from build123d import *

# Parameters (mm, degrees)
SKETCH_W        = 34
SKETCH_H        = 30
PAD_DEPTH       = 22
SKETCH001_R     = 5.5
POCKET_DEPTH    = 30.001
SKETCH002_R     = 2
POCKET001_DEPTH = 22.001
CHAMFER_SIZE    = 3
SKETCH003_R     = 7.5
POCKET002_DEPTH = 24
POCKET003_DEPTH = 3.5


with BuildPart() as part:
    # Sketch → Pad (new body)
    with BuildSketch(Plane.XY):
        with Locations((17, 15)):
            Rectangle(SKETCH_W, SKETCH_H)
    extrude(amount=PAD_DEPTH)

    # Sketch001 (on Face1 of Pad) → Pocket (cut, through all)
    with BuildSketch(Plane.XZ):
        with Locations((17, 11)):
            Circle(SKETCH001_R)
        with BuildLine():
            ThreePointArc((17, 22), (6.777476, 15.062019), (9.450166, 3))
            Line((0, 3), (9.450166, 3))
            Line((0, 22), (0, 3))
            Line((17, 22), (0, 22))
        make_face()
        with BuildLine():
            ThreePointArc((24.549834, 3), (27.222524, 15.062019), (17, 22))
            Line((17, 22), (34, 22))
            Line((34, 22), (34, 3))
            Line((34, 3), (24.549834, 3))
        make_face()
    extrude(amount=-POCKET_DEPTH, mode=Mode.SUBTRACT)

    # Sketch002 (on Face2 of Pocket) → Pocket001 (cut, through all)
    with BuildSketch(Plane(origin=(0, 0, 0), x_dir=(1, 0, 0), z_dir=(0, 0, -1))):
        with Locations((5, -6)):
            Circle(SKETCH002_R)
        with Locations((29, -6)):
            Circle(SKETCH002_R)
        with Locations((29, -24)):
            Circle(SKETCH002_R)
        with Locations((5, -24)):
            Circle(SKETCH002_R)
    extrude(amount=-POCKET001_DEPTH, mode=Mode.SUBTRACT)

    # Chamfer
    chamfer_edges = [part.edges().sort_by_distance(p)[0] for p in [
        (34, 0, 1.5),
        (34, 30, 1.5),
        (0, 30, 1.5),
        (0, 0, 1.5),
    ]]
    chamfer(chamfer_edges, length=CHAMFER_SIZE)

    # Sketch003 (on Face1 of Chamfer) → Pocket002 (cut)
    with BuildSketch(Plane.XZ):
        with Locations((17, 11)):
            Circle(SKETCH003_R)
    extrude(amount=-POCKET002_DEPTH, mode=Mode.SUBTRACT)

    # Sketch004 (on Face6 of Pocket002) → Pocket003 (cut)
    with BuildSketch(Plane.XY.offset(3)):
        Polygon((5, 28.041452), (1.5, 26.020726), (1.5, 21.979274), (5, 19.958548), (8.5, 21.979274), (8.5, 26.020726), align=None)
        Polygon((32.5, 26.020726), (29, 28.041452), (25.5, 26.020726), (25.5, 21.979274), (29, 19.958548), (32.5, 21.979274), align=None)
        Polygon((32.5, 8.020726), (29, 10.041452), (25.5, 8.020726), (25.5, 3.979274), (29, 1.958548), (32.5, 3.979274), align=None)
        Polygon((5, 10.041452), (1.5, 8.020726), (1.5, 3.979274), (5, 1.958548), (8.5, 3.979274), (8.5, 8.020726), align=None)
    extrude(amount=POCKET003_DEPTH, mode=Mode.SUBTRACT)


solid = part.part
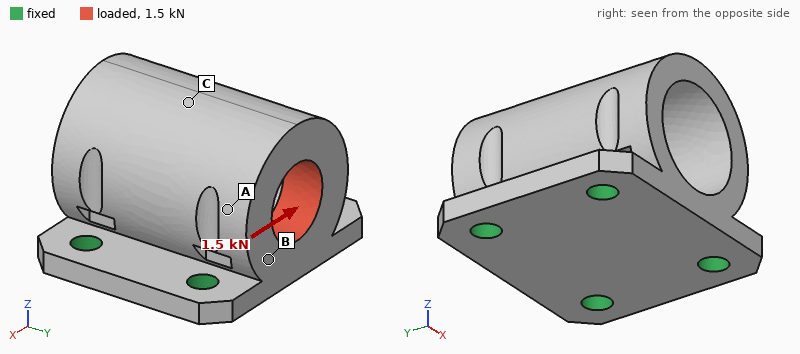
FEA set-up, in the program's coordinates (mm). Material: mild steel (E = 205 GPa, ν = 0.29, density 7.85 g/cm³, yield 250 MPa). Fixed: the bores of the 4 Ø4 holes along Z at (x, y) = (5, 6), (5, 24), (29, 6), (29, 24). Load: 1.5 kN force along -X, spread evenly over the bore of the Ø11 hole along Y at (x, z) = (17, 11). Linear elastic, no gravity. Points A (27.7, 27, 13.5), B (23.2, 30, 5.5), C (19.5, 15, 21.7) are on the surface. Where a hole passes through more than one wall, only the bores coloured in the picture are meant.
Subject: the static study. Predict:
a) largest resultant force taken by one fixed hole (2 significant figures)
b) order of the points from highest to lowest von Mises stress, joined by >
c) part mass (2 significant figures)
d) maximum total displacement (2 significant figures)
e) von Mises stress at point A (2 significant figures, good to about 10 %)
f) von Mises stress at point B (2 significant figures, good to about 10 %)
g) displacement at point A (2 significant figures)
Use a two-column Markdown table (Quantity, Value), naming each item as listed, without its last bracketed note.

| Quantity | Value |
|---|---|
| largest resultant force taken by one fixed hole | 790 N |
| order of the points from highest to lowest von Mises stress, joined by > | B > A > C |
| part mass | 66 g |
| maximum total displacement | 9.9 µm |
| von Mises stress at point A | 17 MPa |
| von Mises stress at point B | 24 MPa |
| displacement at point A | 8.0 µm |
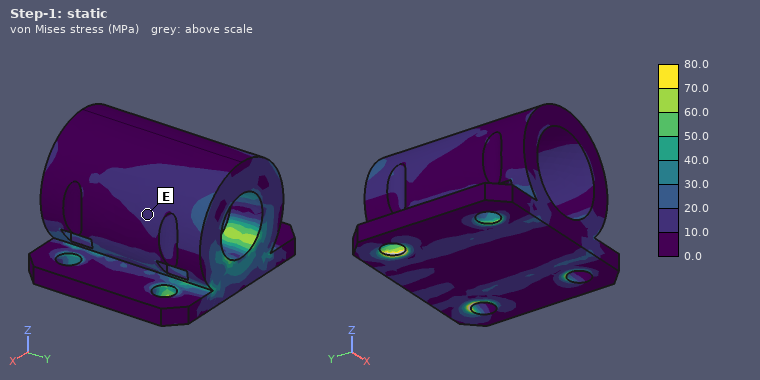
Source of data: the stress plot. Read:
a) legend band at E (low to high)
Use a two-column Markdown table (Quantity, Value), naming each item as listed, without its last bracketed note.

| Quantity | Value |
|---|---|
| legend band at E | 10.0 to 20.0 MPa |
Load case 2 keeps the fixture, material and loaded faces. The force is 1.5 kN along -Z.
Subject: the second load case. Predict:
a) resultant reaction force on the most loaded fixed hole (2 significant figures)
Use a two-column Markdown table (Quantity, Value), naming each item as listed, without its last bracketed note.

| Quantity | Value |
|---|---|
| resultant reaction force on the most loaded fixed hole | 850 N |
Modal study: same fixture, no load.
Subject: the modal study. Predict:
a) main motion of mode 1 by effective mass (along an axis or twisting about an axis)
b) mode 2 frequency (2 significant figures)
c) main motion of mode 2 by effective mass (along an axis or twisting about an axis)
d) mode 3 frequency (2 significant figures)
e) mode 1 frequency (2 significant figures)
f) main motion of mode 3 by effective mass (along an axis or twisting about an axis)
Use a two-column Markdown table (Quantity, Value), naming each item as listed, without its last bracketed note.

| Quantity | Value |
|---|---|
| main motion of mode 1 by effective mass | along X |
| mode 2 frequency | 12 kHz |
| main motion of mode 2 by effective mass | along Y |
| mode 3 frequency | 19 kHz |
| mode 1 frequency | 9600 Hz |
| main motion of mode 3 by effective mass | along Z |
